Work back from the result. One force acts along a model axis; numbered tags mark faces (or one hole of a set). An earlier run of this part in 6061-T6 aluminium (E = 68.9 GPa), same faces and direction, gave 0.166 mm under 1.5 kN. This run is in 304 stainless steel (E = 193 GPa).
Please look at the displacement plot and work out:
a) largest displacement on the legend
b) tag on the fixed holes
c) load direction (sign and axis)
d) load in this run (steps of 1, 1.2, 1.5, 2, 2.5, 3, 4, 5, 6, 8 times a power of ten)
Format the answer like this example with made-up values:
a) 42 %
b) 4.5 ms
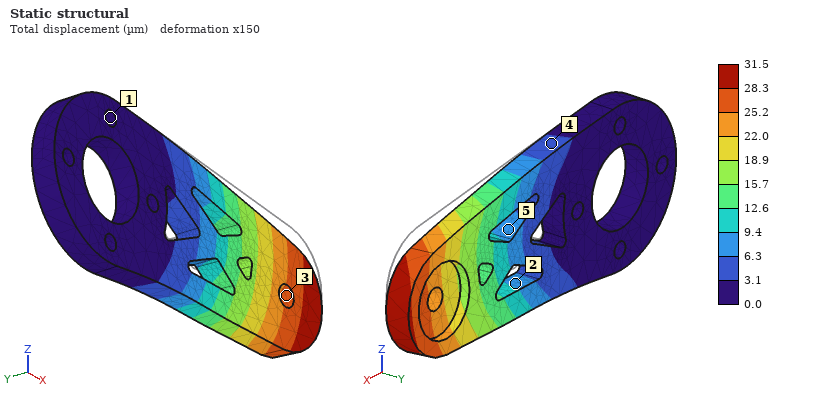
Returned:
a) 31.5 µm
b) 1
c) -Z
d) 800 N
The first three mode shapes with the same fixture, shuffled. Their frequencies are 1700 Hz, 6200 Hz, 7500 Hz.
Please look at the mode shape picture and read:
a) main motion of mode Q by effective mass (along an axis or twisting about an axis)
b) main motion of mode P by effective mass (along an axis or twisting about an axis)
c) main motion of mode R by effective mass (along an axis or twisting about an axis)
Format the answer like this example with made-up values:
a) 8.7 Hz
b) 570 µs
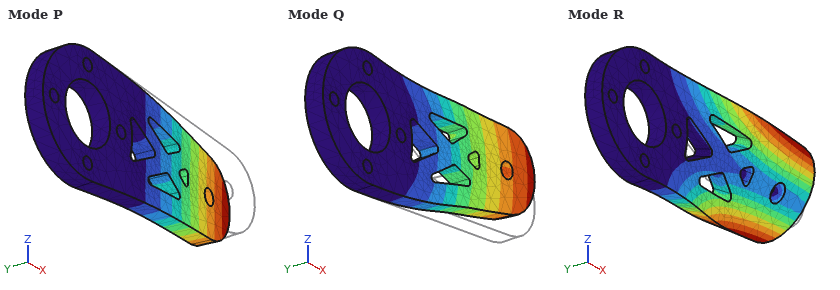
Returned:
a) along Z
b) along Y
c) twisting about X
